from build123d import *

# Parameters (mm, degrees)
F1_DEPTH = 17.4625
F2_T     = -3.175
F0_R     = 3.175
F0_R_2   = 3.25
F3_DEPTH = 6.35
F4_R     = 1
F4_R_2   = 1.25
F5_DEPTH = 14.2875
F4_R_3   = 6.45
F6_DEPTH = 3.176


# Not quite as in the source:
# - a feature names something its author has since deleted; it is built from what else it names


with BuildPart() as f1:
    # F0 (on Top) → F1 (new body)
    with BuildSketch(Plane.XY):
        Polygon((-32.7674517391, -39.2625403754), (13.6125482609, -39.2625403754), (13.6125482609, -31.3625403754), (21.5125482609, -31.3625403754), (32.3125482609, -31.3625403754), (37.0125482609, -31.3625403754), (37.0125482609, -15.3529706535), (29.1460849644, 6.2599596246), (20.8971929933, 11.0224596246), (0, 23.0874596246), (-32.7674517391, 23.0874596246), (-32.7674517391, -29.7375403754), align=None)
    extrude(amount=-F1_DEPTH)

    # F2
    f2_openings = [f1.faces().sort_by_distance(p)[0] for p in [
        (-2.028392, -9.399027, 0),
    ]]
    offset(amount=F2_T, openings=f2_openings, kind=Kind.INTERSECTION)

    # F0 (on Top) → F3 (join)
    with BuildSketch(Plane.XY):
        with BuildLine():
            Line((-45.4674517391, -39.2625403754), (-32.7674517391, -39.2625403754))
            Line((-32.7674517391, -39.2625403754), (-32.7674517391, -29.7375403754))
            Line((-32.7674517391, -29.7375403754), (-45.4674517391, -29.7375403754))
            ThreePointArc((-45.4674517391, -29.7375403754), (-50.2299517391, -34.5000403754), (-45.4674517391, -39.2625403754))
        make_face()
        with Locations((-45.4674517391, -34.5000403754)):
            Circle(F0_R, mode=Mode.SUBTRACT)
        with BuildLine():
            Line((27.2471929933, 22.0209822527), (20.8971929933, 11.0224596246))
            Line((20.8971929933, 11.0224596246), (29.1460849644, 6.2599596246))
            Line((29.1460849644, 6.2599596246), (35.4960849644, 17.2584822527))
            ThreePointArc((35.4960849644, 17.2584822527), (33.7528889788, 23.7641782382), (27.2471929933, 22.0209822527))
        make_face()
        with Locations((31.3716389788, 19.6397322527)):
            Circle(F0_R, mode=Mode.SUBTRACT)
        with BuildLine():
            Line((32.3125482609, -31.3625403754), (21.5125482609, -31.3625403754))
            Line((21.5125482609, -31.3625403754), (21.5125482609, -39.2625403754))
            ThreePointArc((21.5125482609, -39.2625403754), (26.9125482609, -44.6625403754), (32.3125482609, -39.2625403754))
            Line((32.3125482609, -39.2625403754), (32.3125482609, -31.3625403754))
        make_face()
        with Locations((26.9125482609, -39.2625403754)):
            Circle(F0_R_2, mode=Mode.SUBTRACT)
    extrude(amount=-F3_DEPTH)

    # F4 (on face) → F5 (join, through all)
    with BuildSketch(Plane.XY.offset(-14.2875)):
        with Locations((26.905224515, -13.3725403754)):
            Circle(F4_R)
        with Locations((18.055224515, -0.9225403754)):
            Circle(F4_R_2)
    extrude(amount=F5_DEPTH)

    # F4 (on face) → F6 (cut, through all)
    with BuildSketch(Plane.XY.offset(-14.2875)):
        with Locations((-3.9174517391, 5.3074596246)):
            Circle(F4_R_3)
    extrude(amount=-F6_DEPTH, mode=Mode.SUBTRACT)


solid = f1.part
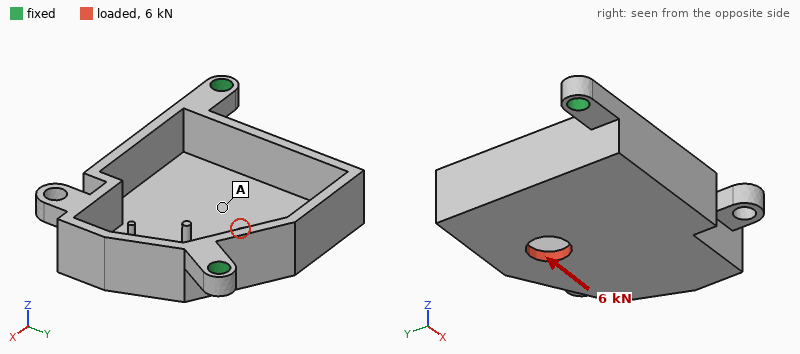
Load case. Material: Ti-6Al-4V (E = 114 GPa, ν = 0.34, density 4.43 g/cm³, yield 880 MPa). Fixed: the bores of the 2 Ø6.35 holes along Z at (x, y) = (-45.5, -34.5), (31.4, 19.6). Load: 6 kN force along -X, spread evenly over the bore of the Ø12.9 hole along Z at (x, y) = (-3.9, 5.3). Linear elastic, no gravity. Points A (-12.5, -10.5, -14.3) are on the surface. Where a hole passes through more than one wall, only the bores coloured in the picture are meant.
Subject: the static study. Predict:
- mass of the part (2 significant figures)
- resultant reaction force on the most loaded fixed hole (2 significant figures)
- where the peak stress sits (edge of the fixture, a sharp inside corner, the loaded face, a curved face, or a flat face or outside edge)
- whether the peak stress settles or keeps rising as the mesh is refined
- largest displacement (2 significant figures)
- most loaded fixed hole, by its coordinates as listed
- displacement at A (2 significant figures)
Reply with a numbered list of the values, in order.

1. 110 g
2. 3.8 kN
3. edge of the fixture
4. keeps rising
5. 0.70 mm
6. (31.4, 19.6)
7. 0.19 mm
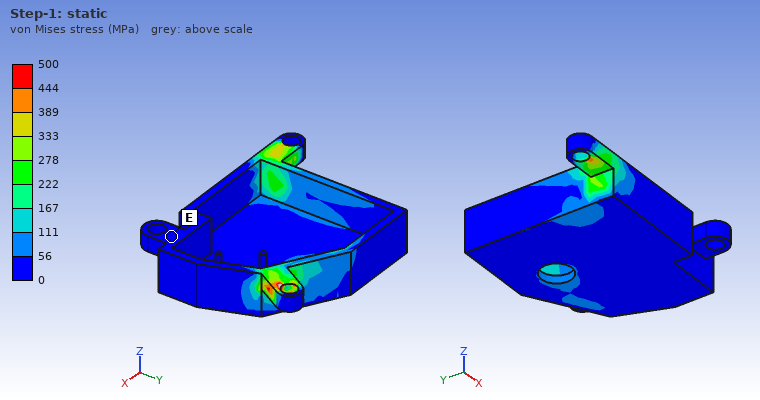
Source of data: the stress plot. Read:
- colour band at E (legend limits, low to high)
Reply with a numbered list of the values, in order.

1. 0 to 56 MPa
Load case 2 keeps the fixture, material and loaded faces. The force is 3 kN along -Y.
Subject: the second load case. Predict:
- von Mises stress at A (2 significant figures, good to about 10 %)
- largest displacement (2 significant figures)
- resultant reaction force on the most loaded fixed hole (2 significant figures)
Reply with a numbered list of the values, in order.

1. 23 MPa
2. 0.48 mm
3. 1.6 kN
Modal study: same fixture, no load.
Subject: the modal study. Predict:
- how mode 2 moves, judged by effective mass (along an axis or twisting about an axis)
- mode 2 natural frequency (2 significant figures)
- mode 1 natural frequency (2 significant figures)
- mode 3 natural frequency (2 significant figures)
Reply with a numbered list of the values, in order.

1. along Z
2. 3100 Hz
3. 1200 Hz
4. 4100 Hz
